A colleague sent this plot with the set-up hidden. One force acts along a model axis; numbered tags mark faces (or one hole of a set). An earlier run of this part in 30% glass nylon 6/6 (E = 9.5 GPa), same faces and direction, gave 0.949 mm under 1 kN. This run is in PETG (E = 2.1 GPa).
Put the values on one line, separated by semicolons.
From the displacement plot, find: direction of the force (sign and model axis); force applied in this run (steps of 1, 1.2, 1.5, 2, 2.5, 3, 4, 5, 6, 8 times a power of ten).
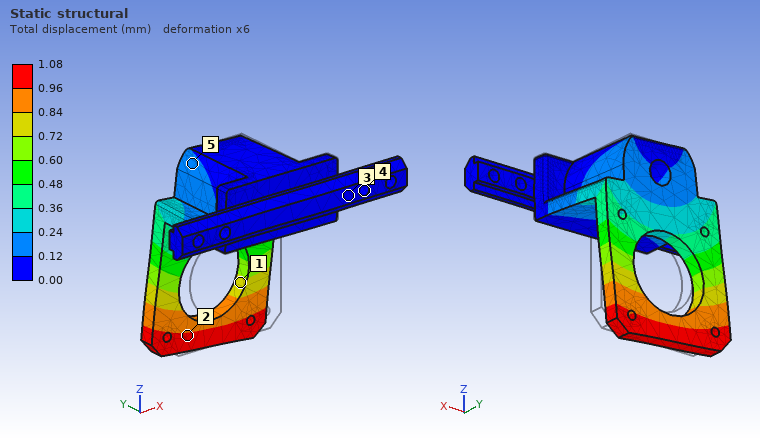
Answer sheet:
-X; 250 N
